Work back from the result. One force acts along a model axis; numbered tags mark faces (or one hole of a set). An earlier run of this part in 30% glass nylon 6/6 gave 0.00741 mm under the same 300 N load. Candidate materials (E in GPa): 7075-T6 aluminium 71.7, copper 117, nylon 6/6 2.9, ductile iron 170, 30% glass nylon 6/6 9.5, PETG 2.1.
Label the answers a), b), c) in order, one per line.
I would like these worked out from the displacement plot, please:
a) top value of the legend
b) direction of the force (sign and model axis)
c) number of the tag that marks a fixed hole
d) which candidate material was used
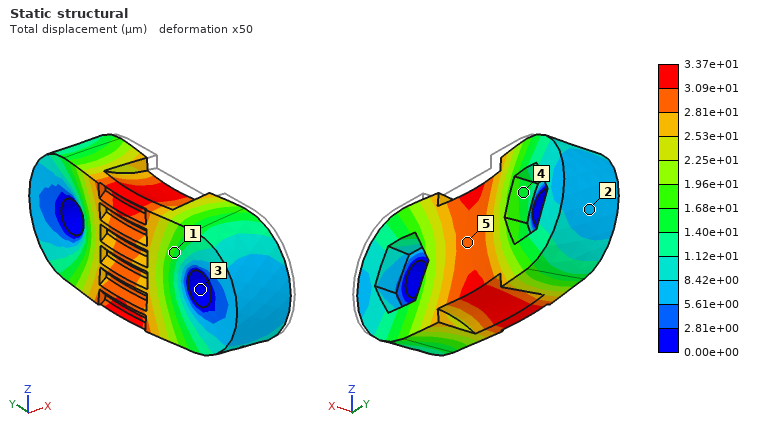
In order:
a) 3.37e+01 µm
b) -X
c) 3
d) PETG
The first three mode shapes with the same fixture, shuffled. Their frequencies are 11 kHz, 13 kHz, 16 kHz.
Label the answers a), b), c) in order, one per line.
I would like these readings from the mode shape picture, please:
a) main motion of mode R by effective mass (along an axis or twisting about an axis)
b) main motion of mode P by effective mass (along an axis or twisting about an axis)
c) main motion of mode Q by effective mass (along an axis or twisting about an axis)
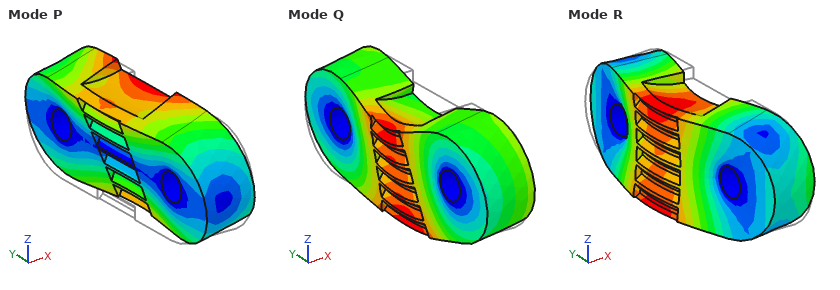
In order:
a) along X
b) along Z
c) along Z
